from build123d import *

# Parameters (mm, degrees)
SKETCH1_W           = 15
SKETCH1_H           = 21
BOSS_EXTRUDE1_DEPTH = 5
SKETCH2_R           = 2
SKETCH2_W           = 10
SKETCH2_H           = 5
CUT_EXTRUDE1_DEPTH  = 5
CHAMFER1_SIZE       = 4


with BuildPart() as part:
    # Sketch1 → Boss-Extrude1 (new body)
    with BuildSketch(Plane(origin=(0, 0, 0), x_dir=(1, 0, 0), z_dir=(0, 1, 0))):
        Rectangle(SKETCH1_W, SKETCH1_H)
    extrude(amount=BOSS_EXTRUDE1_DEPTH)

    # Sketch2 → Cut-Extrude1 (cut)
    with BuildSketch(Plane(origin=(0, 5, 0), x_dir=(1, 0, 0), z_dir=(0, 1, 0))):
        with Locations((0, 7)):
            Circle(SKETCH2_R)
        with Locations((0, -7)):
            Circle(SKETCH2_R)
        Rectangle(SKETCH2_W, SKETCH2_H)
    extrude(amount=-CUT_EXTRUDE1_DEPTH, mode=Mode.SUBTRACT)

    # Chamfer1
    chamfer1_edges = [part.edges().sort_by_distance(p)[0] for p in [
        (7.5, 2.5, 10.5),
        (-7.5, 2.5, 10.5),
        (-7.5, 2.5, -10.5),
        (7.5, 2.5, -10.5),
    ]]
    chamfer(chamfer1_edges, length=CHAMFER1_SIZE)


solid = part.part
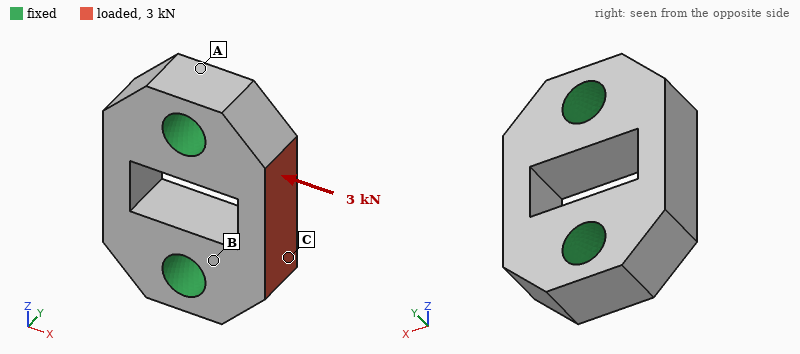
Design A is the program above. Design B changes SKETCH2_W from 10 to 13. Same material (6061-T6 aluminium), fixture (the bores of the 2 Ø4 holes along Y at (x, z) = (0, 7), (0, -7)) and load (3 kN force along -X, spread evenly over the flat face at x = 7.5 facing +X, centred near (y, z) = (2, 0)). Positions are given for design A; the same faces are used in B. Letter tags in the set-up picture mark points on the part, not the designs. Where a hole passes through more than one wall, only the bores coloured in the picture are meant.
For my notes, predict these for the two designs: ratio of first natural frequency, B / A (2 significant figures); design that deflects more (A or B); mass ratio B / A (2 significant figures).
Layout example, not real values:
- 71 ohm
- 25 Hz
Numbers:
- 1.1
- B
- 0.93
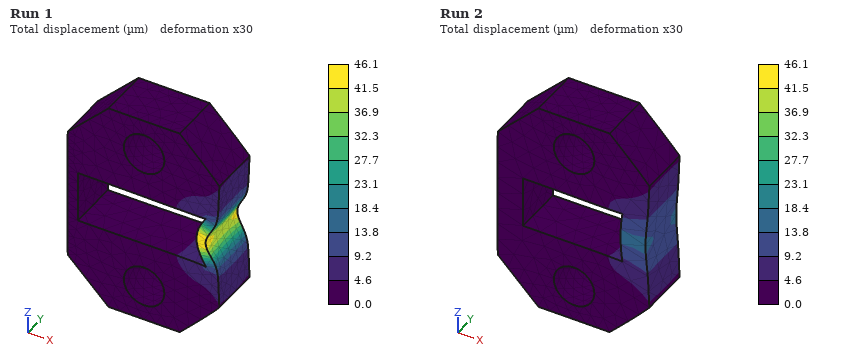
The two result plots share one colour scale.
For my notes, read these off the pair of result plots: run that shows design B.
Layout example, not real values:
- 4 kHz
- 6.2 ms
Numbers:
- Run 1
